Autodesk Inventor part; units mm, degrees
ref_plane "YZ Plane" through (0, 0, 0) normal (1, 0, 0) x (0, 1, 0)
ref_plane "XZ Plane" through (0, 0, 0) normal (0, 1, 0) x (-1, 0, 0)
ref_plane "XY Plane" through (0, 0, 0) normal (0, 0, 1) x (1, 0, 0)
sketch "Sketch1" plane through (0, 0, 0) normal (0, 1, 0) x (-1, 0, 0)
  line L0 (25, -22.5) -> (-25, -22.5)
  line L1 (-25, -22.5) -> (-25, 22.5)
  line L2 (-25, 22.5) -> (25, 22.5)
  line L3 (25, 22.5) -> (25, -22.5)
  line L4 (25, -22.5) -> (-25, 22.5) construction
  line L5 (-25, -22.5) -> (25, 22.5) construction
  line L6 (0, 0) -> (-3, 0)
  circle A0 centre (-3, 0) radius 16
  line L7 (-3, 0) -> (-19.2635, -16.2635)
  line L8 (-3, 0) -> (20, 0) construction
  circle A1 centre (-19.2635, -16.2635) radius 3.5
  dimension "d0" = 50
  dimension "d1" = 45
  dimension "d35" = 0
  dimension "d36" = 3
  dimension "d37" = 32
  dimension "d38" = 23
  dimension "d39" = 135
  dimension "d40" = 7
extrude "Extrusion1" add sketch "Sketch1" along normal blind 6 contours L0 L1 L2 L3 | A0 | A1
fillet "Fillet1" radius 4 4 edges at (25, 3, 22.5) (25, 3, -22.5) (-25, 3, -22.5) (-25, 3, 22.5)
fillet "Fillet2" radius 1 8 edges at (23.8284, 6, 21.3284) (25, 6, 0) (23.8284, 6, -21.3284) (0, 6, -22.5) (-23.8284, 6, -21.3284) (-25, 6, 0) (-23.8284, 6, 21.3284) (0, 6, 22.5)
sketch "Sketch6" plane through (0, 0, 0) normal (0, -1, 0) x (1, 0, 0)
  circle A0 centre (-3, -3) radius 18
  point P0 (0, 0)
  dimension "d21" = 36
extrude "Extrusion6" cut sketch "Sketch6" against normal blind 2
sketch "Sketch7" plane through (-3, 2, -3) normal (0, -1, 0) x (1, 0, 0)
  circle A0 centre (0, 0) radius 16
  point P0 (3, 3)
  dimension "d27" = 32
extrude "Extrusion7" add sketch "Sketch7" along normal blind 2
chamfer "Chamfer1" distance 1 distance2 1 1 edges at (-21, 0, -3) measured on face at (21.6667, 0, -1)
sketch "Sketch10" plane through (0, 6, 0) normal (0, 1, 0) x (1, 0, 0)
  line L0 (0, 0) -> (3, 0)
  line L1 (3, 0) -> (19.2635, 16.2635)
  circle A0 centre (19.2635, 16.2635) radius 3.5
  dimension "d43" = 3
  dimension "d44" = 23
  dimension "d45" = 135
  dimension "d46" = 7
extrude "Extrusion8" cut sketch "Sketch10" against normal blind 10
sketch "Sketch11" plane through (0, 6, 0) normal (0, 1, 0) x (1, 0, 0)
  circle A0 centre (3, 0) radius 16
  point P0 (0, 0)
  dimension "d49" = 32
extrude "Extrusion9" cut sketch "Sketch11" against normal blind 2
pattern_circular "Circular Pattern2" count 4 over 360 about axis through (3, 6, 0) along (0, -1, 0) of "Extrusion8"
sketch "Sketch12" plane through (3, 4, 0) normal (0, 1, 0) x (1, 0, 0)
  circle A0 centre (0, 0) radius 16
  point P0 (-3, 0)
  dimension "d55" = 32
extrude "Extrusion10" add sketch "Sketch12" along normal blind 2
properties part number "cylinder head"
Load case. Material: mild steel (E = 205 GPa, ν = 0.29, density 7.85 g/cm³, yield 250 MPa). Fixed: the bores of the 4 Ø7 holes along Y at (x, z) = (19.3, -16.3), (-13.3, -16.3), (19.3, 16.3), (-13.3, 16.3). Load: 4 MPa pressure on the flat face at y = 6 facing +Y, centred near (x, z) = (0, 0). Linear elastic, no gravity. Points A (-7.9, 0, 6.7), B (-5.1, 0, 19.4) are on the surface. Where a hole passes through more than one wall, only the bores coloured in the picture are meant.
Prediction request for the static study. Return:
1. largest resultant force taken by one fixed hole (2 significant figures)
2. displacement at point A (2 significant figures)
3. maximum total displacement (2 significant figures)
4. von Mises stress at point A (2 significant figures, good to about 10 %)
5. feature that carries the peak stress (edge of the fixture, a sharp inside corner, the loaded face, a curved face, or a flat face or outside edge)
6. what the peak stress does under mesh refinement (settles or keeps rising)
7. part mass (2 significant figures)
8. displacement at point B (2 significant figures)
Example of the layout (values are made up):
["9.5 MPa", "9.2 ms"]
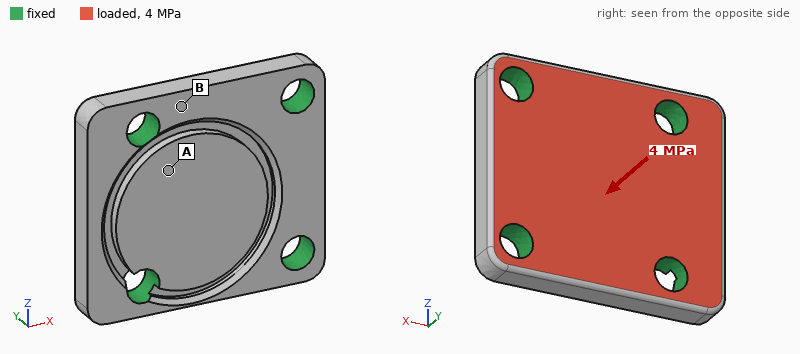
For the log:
["2.2 kN", "4.3 µm", "6.7 µm", "23 MPa", "edge of the fixture", "keeps rising", "94 g", "1.6 µm"]
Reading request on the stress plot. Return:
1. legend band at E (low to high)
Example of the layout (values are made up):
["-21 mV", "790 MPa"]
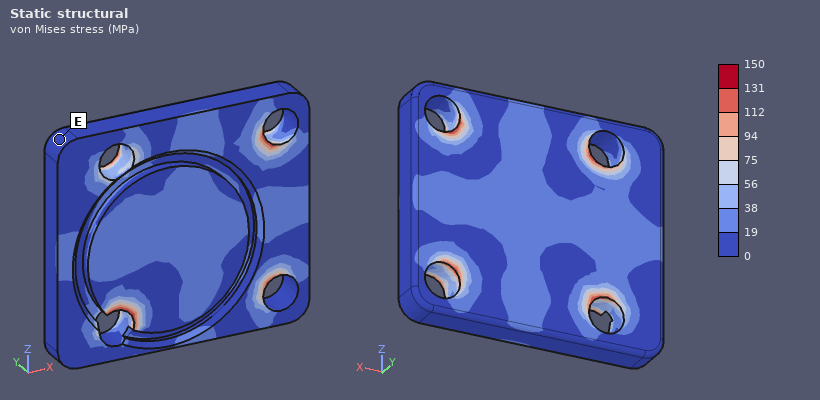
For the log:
["0 to 19 MPa"]
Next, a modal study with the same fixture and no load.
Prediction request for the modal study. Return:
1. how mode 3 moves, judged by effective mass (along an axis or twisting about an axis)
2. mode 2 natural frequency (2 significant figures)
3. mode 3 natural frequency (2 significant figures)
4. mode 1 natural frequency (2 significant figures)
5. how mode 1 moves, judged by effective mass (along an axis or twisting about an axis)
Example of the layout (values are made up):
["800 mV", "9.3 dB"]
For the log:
["twisting about X", "25 kHz", "33 kHz", "22 kHz", "along Y"]
